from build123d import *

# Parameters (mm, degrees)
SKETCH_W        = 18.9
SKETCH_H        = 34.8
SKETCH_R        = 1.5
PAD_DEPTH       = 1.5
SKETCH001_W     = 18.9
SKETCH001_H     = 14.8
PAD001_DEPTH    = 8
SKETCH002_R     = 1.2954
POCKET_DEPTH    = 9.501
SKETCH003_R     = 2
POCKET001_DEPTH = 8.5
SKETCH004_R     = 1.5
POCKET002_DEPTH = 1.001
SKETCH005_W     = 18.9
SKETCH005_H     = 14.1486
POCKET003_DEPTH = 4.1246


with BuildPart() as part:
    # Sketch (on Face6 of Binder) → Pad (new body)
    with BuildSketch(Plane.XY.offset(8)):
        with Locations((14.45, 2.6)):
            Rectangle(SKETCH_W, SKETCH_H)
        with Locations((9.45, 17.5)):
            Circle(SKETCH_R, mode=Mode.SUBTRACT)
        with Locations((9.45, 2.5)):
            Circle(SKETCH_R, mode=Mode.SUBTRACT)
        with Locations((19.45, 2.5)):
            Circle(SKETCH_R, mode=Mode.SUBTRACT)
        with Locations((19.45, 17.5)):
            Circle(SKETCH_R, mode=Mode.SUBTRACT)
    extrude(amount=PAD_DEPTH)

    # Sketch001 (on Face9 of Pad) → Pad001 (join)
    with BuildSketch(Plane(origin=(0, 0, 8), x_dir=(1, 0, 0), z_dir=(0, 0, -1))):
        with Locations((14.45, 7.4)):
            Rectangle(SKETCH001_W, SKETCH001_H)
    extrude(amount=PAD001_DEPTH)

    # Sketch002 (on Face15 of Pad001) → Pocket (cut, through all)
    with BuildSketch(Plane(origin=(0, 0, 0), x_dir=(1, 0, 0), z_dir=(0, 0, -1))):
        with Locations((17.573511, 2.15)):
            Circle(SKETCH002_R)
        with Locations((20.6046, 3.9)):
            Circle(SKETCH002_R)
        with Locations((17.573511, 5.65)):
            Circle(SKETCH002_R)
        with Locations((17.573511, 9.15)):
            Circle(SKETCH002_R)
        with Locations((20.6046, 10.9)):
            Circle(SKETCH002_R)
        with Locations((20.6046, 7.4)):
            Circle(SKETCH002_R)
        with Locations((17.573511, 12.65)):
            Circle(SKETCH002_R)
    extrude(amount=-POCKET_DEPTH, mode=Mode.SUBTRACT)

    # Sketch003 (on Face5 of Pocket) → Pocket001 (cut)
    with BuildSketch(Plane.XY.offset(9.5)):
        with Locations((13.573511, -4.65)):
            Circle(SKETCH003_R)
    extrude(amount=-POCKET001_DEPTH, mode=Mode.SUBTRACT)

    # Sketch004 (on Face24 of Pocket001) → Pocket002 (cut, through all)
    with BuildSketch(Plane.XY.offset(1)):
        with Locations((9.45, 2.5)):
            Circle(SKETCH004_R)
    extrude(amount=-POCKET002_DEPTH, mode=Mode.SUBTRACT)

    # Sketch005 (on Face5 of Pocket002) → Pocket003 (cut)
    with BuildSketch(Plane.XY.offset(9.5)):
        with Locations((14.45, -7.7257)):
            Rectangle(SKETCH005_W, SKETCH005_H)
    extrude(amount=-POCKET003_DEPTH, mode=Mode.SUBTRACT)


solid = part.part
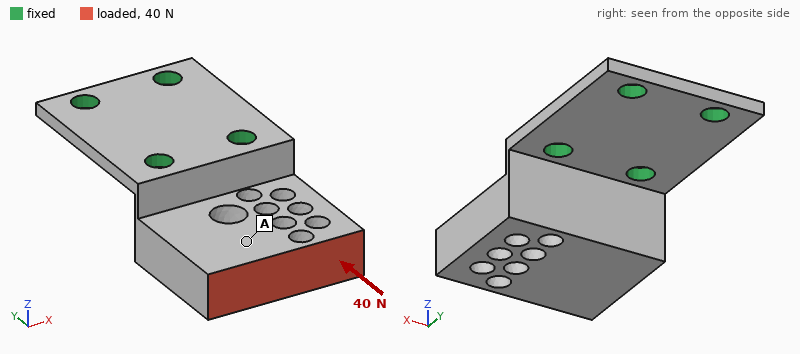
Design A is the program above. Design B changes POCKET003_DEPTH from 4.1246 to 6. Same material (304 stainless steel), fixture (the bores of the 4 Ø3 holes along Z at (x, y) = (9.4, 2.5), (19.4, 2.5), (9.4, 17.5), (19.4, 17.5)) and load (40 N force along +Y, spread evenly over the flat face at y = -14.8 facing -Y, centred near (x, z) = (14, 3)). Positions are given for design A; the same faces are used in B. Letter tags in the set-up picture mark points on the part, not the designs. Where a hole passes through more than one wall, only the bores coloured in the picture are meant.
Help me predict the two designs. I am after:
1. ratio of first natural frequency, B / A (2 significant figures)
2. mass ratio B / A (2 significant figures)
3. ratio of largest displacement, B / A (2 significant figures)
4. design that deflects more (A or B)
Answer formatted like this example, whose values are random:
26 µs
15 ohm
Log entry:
0.99
0.78
1.6
B
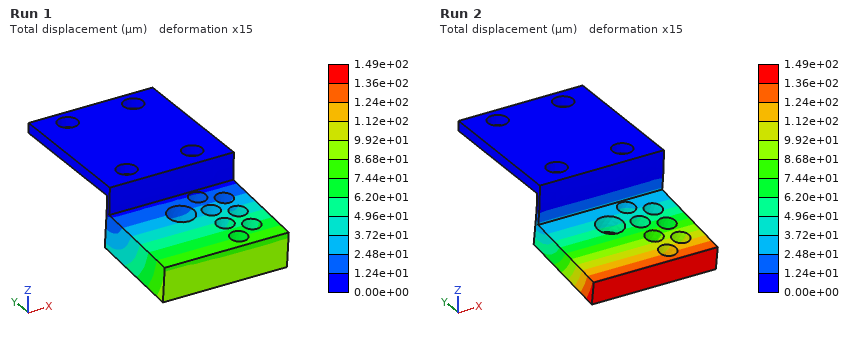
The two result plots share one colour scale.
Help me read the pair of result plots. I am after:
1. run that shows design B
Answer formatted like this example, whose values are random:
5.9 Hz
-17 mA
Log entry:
Run 2
